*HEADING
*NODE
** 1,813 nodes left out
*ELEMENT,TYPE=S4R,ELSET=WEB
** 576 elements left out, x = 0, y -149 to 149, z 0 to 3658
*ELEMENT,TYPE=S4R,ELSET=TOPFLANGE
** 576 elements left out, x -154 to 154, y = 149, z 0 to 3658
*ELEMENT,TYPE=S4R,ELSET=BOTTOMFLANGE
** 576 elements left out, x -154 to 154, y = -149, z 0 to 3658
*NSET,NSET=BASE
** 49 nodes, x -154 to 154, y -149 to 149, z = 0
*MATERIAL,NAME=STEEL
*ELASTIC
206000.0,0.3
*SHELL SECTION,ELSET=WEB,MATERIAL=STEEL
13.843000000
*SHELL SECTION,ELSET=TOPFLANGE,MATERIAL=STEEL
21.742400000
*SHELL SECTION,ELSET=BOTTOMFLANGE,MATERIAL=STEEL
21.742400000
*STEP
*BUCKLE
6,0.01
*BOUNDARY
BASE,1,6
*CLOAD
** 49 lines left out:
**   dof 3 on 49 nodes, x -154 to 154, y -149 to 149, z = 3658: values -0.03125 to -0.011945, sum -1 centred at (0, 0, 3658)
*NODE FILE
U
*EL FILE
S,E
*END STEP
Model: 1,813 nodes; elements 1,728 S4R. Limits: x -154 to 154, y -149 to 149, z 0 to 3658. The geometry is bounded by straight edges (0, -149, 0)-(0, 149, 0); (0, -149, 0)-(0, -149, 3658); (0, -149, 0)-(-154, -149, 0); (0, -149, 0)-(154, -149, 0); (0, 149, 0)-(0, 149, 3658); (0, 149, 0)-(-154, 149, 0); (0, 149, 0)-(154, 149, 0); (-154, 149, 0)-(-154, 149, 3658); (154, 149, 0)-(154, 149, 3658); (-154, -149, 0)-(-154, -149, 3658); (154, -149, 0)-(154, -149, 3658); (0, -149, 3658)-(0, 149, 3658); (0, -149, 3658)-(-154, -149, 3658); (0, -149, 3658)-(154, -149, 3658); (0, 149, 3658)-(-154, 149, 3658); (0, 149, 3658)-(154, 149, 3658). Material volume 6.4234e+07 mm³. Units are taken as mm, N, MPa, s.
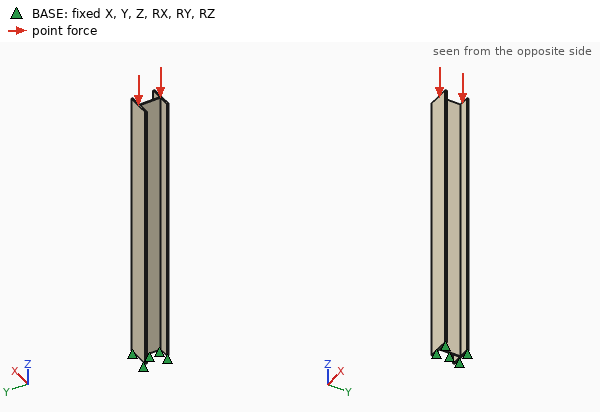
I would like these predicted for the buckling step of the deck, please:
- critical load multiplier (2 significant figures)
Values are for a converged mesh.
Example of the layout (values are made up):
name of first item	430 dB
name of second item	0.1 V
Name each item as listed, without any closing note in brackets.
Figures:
critical load multiplier	4.0e+06
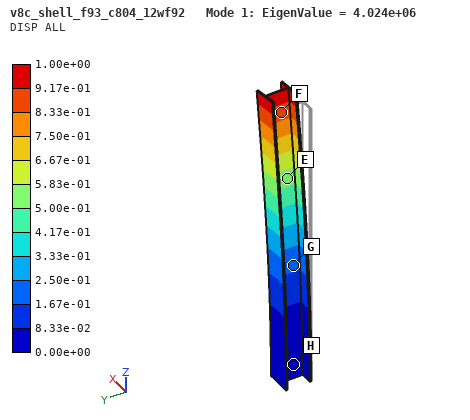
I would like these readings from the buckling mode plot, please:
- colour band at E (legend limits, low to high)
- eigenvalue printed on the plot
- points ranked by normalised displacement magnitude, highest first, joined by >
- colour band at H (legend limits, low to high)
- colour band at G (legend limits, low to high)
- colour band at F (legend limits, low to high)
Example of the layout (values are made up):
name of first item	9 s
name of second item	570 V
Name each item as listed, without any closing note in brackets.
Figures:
colour band at E	5.00e-01 to 5.83e-01
eigenvalue printed on the plot	4.024e+06
points ranked by normalised displacement magnitude, highest first, joined by >	F > E > G > H
colour band at H	0.00e+00 to 8.33e-02
colour band at G	1.67e-01 to 2.50e-01
colour band at F	8.33e-01 to 9.17e-01
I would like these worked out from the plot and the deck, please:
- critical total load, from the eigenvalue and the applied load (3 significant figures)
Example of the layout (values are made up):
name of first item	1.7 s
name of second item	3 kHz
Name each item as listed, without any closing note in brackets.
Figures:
critical total load, from the eigenvalue and the applied load	4.02e+06 N
